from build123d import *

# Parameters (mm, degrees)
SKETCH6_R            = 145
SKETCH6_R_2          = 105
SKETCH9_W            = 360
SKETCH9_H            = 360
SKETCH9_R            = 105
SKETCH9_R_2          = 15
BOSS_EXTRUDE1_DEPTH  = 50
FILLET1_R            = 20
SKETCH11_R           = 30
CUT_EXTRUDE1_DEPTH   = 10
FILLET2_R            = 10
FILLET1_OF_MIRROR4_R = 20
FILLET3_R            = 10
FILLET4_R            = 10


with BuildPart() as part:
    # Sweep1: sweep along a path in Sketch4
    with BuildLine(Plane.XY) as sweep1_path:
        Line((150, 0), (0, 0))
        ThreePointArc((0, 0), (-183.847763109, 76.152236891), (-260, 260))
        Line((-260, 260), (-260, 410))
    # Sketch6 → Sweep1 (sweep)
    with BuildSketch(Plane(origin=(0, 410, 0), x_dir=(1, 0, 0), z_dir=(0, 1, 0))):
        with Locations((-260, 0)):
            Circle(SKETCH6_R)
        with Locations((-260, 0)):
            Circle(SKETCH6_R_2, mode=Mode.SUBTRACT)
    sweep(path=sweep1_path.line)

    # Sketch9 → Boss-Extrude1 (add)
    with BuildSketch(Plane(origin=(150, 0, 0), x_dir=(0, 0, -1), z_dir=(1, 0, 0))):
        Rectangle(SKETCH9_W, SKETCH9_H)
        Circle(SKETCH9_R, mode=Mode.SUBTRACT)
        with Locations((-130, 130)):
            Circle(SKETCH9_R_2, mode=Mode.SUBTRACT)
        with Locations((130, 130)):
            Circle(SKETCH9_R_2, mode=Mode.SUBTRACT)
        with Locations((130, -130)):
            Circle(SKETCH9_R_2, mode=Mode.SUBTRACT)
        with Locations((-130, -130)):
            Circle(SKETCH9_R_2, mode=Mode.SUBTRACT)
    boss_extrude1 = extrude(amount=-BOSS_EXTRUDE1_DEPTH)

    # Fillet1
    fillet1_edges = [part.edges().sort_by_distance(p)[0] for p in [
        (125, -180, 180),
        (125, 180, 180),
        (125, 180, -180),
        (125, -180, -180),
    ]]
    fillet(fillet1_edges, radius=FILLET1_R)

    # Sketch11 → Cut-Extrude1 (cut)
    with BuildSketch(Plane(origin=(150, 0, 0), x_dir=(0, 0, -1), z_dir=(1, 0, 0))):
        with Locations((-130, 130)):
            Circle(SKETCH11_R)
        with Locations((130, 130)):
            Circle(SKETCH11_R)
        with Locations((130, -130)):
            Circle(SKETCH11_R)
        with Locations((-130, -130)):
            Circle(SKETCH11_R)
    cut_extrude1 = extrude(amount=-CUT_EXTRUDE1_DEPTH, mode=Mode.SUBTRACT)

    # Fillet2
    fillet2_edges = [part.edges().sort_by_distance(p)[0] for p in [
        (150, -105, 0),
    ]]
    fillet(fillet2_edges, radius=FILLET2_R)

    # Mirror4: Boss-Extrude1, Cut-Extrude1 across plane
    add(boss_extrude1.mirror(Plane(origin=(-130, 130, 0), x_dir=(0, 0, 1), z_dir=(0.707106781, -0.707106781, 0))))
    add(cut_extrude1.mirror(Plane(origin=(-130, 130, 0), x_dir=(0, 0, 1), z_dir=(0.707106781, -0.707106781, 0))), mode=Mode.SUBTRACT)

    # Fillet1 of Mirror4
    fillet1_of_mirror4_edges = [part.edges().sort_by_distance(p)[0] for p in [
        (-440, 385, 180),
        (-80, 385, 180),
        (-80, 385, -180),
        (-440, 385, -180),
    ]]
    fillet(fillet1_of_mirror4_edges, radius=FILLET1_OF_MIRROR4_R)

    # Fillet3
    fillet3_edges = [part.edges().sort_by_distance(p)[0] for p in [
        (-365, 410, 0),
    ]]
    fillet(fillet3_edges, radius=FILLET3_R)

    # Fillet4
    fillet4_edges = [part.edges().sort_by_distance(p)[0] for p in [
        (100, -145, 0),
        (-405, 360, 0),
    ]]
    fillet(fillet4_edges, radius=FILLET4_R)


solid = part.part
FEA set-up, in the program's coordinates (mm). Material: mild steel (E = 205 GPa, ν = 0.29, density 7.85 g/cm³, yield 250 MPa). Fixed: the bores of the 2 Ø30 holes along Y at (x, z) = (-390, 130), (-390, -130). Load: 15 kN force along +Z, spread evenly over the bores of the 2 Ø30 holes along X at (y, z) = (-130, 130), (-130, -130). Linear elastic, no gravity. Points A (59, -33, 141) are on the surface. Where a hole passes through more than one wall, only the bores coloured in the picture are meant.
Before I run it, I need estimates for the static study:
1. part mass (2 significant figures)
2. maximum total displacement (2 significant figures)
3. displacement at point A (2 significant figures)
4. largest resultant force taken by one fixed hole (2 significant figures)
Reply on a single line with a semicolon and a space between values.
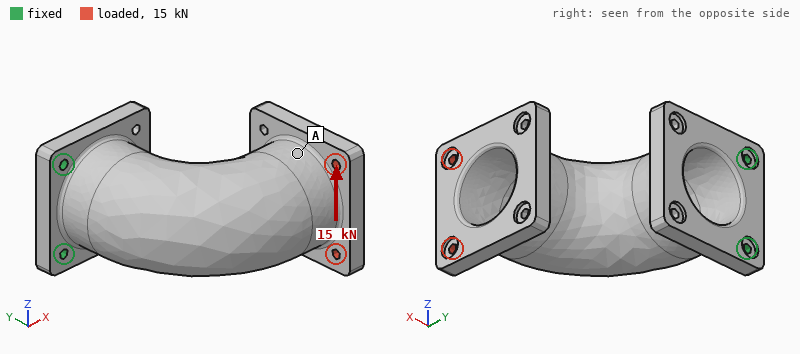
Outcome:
220 kg; 0.12 mm; 0.089 mm; 42 kN
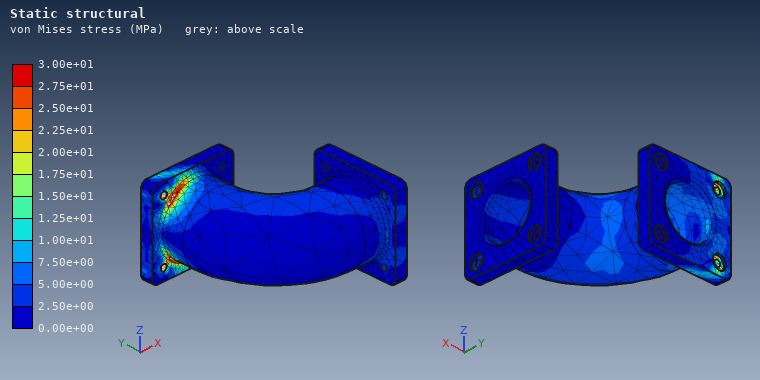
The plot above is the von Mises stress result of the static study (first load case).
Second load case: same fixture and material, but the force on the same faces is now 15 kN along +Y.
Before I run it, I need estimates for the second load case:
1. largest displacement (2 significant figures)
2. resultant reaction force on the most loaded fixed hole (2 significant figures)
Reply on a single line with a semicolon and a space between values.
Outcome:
0.75 mm; 7.6 kN
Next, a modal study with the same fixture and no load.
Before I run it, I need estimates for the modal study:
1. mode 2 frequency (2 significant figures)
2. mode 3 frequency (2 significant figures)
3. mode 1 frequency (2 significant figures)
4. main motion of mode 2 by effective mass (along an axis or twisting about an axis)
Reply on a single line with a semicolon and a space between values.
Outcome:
230 Hz; 550 Hz; 70 Hz; along Z
